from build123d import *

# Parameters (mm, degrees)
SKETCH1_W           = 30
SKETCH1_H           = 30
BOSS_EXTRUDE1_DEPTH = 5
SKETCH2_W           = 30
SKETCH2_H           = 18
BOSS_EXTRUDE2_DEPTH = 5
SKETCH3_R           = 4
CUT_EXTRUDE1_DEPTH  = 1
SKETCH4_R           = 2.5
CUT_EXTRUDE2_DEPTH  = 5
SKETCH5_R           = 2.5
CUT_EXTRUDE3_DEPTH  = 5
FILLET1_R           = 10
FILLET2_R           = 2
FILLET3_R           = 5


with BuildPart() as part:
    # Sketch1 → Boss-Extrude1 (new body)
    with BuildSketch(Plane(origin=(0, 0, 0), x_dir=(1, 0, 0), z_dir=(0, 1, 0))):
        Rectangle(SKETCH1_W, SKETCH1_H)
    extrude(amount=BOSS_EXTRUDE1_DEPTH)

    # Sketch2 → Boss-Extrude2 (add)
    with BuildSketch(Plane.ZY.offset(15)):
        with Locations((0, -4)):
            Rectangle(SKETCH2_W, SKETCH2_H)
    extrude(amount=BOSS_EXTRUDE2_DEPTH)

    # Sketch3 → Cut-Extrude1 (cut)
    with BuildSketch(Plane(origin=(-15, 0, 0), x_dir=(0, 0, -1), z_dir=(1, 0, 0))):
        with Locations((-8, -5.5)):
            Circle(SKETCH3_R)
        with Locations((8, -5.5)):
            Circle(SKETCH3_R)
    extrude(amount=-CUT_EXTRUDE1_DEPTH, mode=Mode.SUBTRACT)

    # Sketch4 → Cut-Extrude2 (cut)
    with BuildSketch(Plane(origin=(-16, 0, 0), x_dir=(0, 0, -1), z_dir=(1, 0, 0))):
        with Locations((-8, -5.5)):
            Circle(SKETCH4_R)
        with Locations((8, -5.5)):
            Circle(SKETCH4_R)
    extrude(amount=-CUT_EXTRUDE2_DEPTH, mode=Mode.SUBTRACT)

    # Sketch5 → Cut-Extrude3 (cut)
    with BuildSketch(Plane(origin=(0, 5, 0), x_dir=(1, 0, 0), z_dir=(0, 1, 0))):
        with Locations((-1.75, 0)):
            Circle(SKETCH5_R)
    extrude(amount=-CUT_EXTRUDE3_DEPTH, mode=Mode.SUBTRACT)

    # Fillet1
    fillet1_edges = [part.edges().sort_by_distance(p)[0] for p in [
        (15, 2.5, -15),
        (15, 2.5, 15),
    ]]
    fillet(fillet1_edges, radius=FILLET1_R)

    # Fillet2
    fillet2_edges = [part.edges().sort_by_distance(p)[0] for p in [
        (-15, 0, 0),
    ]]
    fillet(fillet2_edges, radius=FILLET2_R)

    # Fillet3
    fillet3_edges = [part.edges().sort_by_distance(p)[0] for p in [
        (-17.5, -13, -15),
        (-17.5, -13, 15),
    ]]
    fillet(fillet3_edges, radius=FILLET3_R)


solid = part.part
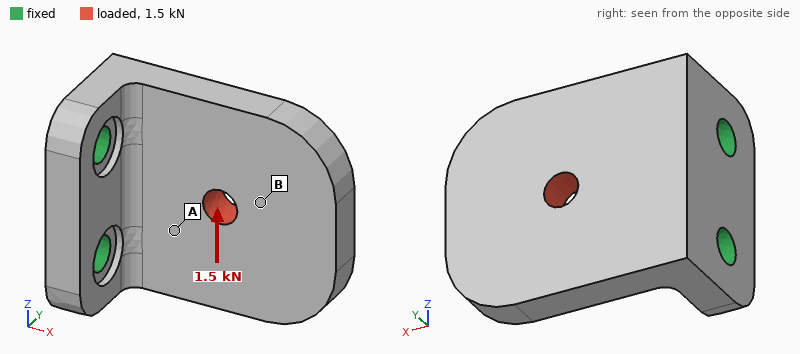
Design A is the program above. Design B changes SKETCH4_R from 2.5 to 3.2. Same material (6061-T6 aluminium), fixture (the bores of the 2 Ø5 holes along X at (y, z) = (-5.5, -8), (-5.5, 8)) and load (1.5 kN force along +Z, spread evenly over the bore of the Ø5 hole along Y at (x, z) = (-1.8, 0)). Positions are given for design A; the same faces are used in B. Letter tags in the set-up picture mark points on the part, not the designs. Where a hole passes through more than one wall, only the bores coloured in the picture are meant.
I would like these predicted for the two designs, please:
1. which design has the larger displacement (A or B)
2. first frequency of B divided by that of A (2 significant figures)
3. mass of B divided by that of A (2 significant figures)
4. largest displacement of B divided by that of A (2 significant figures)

A
1.1
0.98
0.81
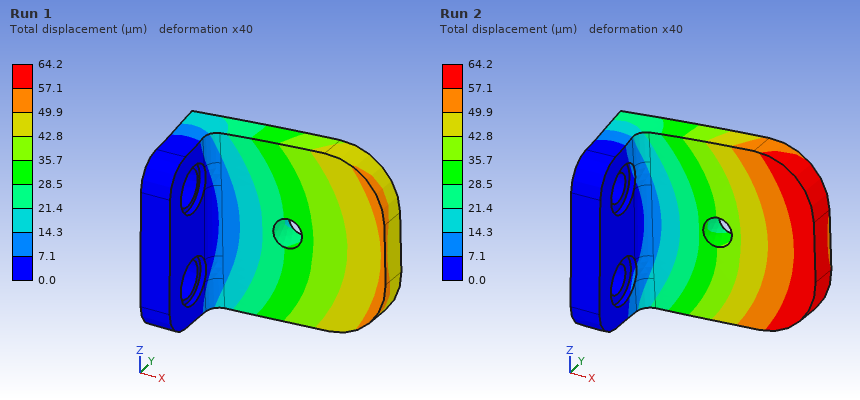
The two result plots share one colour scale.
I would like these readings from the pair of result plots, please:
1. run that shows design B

Run 1
